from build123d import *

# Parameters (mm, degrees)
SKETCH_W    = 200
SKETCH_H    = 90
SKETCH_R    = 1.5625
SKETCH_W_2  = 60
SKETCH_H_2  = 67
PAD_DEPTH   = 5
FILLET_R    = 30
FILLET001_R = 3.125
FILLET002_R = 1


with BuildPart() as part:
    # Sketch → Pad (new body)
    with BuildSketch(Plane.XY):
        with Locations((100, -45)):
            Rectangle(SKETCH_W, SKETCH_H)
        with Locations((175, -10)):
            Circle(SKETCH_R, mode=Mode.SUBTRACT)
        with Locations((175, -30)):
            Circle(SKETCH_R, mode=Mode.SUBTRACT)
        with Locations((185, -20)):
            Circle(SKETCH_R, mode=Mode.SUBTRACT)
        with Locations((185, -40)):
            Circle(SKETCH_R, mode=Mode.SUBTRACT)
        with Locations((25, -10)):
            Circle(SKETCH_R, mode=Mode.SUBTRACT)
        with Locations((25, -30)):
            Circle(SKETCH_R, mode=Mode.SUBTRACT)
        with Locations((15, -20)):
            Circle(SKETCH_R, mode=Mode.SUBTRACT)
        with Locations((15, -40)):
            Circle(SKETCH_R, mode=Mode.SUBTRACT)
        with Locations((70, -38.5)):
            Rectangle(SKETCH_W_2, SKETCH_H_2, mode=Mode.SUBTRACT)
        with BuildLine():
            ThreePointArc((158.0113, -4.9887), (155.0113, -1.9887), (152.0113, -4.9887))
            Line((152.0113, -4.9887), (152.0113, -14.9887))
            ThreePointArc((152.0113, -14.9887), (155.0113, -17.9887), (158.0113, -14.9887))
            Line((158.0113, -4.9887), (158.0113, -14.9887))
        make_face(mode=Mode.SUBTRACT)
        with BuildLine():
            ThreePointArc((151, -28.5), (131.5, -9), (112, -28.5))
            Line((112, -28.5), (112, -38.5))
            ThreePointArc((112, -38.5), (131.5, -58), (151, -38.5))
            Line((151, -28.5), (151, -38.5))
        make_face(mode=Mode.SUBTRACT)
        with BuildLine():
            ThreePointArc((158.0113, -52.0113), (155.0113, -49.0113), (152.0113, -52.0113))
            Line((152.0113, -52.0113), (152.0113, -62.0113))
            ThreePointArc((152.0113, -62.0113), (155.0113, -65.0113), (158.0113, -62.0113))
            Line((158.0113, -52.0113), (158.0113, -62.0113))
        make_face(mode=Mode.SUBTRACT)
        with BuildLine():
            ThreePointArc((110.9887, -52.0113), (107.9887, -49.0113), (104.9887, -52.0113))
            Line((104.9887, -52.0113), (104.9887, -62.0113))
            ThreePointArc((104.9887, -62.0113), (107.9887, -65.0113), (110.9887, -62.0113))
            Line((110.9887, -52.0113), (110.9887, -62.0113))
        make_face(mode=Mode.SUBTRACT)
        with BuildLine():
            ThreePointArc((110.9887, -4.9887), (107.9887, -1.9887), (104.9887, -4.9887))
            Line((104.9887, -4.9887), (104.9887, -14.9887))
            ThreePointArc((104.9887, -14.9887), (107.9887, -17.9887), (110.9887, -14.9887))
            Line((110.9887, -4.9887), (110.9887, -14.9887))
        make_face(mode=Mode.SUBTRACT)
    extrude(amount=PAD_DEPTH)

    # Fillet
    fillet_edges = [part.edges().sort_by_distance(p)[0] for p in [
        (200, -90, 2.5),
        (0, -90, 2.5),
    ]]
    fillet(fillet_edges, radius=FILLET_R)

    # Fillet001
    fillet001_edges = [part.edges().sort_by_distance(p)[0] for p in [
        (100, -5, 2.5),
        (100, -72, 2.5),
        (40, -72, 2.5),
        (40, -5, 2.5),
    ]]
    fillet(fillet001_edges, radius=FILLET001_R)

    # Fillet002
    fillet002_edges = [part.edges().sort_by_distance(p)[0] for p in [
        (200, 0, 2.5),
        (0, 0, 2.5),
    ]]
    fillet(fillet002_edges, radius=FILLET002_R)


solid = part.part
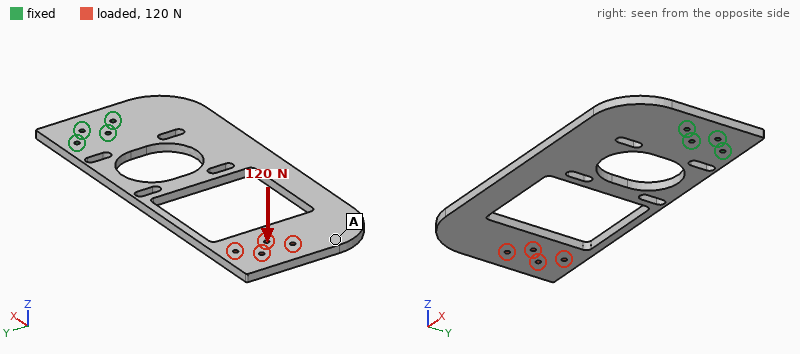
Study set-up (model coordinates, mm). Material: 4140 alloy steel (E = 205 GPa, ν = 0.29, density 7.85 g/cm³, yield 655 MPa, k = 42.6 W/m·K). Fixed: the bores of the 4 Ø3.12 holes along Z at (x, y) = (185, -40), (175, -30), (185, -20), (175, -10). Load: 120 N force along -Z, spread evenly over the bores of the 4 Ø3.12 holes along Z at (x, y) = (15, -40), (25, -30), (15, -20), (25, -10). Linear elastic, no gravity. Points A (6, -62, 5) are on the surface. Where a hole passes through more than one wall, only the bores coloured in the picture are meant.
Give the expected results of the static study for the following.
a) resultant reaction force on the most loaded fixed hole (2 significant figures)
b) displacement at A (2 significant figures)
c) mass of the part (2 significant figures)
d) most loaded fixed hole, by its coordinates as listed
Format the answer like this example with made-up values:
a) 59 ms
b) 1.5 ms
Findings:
a) 780 N
b) 2.3 mm
c) 460 g
d) (175, -30)
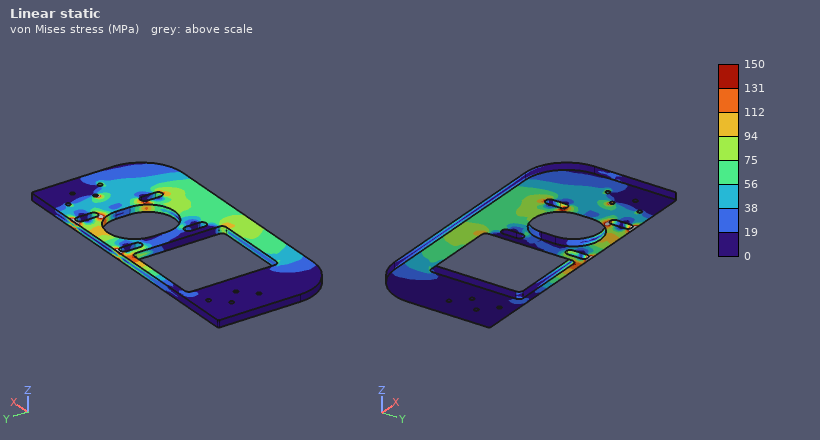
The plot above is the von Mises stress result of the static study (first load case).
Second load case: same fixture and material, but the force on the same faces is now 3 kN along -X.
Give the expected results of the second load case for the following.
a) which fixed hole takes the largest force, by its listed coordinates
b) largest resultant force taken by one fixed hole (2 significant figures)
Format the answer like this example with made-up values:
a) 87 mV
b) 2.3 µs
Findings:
a) (175, -10)
b) 1.3 kN
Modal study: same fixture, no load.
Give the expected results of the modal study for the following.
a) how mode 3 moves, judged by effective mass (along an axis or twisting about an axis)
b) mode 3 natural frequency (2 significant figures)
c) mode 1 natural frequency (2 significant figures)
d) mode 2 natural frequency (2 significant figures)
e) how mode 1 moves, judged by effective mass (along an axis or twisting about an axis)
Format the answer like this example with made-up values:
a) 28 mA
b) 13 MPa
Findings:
a) along Z
b) 660 Hz
c) 100 Hz
d) 370 Hz
e) along Z
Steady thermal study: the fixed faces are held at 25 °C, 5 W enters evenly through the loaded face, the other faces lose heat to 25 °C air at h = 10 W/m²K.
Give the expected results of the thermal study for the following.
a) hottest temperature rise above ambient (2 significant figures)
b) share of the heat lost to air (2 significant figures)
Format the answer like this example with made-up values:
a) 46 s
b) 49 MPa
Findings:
a) 45 K
b) 85 %
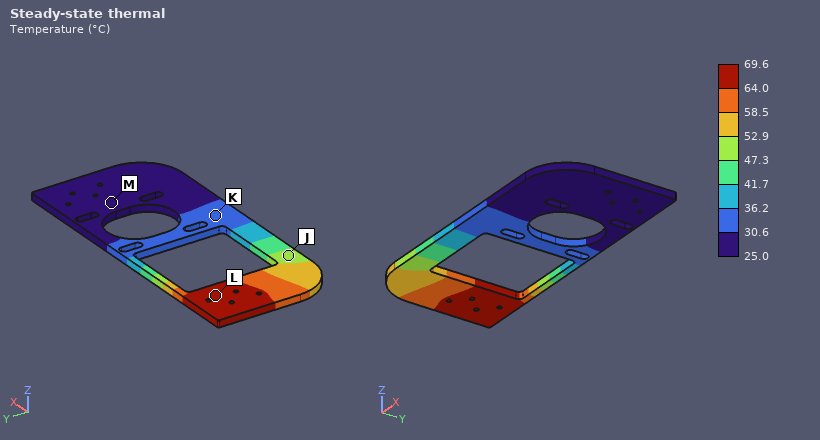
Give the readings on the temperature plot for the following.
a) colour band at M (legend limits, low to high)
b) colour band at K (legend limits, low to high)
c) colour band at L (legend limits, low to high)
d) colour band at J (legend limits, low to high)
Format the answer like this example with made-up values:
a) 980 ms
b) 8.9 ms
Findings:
a) 25.0 to 30.6 °C
b) 30.6 to 36.2 °C
c) 64.0 to 69.6 °C
d) 47.3 to 52.9 °C
